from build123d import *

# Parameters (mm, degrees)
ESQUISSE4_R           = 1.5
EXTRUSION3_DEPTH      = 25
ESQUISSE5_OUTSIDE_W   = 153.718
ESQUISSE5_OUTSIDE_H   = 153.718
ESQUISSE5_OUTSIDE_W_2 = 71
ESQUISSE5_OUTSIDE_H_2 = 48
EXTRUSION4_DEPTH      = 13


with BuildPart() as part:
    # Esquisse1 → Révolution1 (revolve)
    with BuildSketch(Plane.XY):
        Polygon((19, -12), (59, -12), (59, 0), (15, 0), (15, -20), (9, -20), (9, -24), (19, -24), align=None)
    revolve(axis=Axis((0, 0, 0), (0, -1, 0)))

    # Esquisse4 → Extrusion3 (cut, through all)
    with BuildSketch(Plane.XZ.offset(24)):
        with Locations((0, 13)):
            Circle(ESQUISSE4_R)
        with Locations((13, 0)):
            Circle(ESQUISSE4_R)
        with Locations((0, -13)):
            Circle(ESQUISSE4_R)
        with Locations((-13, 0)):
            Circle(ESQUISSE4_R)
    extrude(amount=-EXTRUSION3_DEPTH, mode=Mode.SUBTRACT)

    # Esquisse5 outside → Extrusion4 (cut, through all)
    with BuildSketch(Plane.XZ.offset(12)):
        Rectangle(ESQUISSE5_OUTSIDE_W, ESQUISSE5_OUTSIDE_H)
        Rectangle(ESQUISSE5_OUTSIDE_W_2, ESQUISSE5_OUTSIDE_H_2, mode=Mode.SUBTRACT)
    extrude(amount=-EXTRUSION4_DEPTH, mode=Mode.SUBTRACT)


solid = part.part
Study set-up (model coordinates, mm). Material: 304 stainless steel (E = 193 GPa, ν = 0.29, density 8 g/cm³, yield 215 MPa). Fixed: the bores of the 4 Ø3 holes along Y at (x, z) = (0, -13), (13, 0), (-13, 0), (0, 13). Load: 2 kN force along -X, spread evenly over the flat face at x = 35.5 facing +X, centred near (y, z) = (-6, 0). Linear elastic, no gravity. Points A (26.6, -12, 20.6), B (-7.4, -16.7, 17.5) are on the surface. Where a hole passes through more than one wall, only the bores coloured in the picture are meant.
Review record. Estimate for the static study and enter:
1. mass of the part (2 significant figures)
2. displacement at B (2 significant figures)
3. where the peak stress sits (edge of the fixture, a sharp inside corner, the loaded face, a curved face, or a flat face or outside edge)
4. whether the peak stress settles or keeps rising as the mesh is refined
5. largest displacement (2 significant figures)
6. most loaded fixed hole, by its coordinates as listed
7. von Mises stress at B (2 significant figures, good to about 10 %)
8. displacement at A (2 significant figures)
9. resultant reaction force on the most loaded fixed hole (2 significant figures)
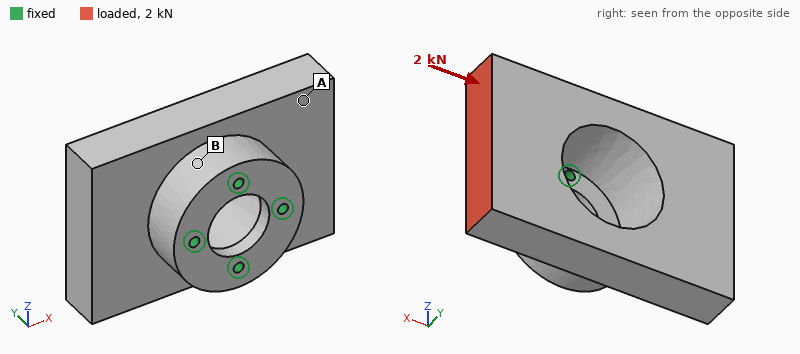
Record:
310 g
2.4 µm
edge of the fixture
keeps rising
9.9 µm
(13, 0)
11 MPa
6.4 µm
1.0 kN
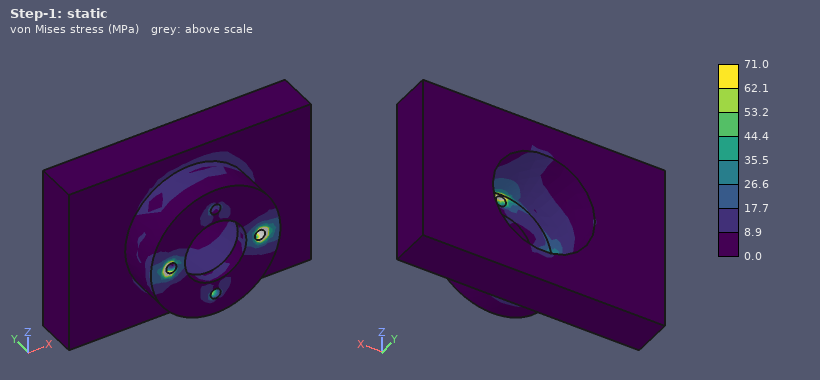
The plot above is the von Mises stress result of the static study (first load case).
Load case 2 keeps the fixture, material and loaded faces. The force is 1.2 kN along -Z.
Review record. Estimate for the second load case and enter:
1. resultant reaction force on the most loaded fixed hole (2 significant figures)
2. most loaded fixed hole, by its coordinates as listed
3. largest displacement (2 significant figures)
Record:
1.3 kN
(13, 0)
8.6 µm
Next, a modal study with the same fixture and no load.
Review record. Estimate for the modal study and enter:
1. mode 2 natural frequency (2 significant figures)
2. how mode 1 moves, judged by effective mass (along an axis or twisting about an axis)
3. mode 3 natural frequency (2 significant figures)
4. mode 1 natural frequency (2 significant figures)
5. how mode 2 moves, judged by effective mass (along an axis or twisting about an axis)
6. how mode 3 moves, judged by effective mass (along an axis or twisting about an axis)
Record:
5300 Hz
along X
7700 Hz
4500 Hz
along Z
twisting about Y
